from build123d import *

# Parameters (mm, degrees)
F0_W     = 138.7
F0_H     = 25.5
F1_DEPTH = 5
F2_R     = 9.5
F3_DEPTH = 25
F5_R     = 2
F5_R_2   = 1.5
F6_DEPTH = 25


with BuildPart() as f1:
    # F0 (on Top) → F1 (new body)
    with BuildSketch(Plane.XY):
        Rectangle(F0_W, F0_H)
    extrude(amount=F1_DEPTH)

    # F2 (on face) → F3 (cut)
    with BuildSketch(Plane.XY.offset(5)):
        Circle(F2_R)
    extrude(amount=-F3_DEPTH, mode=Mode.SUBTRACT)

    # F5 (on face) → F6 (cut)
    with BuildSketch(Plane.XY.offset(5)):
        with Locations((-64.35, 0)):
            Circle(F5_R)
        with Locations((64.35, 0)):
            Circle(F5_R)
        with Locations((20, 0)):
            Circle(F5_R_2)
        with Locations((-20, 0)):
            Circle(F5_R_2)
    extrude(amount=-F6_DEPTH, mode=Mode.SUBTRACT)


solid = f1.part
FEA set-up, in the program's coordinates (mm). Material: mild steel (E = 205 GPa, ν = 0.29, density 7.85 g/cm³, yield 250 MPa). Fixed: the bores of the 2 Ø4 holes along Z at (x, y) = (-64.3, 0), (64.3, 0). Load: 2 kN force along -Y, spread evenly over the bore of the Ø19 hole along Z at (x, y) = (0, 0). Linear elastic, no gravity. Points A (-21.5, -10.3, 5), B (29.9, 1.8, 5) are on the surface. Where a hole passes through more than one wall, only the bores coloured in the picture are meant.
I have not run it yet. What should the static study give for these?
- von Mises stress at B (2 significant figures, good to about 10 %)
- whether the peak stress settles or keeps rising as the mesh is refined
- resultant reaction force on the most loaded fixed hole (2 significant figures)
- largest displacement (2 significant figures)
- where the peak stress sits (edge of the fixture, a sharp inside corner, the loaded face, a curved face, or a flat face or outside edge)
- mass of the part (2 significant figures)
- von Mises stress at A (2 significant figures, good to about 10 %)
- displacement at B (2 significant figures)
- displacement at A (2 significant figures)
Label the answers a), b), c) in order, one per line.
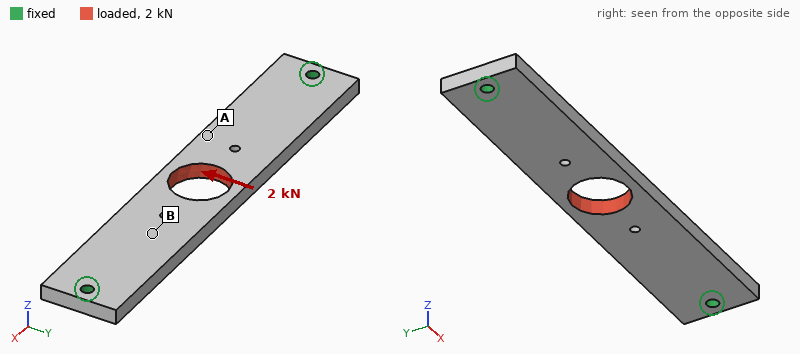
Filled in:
a) 21 MPa
b) keeps rising
c) 1.0 kN
d) 51 µm
e) edge of the fixture
f) 130 g
g) 40 MPa
h) 35 µm
i) 42 µm
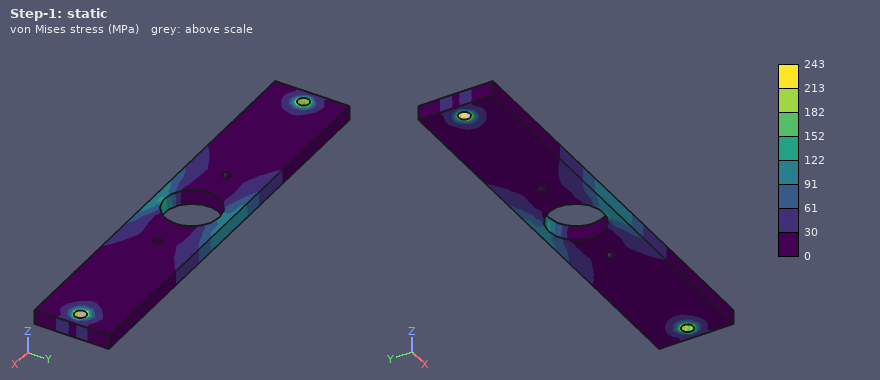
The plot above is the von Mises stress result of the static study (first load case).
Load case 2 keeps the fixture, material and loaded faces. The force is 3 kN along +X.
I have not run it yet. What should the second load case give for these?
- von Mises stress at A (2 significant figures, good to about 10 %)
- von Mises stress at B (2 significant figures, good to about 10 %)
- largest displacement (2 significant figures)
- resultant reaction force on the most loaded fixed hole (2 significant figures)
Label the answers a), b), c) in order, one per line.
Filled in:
a) 12 MPa
b) 11 MPa
c) 4.4 µm
d) 1.5 kN
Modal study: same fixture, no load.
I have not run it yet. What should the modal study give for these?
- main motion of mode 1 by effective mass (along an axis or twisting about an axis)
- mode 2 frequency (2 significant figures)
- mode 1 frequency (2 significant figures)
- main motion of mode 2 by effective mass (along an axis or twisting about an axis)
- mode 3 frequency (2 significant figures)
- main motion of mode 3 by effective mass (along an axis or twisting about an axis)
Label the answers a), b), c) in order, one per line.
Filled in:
a) along Z
b) 4000 Hz
c) 1500 Hz
d) twisting about Y
e) 4400 Hz
f) along Y
